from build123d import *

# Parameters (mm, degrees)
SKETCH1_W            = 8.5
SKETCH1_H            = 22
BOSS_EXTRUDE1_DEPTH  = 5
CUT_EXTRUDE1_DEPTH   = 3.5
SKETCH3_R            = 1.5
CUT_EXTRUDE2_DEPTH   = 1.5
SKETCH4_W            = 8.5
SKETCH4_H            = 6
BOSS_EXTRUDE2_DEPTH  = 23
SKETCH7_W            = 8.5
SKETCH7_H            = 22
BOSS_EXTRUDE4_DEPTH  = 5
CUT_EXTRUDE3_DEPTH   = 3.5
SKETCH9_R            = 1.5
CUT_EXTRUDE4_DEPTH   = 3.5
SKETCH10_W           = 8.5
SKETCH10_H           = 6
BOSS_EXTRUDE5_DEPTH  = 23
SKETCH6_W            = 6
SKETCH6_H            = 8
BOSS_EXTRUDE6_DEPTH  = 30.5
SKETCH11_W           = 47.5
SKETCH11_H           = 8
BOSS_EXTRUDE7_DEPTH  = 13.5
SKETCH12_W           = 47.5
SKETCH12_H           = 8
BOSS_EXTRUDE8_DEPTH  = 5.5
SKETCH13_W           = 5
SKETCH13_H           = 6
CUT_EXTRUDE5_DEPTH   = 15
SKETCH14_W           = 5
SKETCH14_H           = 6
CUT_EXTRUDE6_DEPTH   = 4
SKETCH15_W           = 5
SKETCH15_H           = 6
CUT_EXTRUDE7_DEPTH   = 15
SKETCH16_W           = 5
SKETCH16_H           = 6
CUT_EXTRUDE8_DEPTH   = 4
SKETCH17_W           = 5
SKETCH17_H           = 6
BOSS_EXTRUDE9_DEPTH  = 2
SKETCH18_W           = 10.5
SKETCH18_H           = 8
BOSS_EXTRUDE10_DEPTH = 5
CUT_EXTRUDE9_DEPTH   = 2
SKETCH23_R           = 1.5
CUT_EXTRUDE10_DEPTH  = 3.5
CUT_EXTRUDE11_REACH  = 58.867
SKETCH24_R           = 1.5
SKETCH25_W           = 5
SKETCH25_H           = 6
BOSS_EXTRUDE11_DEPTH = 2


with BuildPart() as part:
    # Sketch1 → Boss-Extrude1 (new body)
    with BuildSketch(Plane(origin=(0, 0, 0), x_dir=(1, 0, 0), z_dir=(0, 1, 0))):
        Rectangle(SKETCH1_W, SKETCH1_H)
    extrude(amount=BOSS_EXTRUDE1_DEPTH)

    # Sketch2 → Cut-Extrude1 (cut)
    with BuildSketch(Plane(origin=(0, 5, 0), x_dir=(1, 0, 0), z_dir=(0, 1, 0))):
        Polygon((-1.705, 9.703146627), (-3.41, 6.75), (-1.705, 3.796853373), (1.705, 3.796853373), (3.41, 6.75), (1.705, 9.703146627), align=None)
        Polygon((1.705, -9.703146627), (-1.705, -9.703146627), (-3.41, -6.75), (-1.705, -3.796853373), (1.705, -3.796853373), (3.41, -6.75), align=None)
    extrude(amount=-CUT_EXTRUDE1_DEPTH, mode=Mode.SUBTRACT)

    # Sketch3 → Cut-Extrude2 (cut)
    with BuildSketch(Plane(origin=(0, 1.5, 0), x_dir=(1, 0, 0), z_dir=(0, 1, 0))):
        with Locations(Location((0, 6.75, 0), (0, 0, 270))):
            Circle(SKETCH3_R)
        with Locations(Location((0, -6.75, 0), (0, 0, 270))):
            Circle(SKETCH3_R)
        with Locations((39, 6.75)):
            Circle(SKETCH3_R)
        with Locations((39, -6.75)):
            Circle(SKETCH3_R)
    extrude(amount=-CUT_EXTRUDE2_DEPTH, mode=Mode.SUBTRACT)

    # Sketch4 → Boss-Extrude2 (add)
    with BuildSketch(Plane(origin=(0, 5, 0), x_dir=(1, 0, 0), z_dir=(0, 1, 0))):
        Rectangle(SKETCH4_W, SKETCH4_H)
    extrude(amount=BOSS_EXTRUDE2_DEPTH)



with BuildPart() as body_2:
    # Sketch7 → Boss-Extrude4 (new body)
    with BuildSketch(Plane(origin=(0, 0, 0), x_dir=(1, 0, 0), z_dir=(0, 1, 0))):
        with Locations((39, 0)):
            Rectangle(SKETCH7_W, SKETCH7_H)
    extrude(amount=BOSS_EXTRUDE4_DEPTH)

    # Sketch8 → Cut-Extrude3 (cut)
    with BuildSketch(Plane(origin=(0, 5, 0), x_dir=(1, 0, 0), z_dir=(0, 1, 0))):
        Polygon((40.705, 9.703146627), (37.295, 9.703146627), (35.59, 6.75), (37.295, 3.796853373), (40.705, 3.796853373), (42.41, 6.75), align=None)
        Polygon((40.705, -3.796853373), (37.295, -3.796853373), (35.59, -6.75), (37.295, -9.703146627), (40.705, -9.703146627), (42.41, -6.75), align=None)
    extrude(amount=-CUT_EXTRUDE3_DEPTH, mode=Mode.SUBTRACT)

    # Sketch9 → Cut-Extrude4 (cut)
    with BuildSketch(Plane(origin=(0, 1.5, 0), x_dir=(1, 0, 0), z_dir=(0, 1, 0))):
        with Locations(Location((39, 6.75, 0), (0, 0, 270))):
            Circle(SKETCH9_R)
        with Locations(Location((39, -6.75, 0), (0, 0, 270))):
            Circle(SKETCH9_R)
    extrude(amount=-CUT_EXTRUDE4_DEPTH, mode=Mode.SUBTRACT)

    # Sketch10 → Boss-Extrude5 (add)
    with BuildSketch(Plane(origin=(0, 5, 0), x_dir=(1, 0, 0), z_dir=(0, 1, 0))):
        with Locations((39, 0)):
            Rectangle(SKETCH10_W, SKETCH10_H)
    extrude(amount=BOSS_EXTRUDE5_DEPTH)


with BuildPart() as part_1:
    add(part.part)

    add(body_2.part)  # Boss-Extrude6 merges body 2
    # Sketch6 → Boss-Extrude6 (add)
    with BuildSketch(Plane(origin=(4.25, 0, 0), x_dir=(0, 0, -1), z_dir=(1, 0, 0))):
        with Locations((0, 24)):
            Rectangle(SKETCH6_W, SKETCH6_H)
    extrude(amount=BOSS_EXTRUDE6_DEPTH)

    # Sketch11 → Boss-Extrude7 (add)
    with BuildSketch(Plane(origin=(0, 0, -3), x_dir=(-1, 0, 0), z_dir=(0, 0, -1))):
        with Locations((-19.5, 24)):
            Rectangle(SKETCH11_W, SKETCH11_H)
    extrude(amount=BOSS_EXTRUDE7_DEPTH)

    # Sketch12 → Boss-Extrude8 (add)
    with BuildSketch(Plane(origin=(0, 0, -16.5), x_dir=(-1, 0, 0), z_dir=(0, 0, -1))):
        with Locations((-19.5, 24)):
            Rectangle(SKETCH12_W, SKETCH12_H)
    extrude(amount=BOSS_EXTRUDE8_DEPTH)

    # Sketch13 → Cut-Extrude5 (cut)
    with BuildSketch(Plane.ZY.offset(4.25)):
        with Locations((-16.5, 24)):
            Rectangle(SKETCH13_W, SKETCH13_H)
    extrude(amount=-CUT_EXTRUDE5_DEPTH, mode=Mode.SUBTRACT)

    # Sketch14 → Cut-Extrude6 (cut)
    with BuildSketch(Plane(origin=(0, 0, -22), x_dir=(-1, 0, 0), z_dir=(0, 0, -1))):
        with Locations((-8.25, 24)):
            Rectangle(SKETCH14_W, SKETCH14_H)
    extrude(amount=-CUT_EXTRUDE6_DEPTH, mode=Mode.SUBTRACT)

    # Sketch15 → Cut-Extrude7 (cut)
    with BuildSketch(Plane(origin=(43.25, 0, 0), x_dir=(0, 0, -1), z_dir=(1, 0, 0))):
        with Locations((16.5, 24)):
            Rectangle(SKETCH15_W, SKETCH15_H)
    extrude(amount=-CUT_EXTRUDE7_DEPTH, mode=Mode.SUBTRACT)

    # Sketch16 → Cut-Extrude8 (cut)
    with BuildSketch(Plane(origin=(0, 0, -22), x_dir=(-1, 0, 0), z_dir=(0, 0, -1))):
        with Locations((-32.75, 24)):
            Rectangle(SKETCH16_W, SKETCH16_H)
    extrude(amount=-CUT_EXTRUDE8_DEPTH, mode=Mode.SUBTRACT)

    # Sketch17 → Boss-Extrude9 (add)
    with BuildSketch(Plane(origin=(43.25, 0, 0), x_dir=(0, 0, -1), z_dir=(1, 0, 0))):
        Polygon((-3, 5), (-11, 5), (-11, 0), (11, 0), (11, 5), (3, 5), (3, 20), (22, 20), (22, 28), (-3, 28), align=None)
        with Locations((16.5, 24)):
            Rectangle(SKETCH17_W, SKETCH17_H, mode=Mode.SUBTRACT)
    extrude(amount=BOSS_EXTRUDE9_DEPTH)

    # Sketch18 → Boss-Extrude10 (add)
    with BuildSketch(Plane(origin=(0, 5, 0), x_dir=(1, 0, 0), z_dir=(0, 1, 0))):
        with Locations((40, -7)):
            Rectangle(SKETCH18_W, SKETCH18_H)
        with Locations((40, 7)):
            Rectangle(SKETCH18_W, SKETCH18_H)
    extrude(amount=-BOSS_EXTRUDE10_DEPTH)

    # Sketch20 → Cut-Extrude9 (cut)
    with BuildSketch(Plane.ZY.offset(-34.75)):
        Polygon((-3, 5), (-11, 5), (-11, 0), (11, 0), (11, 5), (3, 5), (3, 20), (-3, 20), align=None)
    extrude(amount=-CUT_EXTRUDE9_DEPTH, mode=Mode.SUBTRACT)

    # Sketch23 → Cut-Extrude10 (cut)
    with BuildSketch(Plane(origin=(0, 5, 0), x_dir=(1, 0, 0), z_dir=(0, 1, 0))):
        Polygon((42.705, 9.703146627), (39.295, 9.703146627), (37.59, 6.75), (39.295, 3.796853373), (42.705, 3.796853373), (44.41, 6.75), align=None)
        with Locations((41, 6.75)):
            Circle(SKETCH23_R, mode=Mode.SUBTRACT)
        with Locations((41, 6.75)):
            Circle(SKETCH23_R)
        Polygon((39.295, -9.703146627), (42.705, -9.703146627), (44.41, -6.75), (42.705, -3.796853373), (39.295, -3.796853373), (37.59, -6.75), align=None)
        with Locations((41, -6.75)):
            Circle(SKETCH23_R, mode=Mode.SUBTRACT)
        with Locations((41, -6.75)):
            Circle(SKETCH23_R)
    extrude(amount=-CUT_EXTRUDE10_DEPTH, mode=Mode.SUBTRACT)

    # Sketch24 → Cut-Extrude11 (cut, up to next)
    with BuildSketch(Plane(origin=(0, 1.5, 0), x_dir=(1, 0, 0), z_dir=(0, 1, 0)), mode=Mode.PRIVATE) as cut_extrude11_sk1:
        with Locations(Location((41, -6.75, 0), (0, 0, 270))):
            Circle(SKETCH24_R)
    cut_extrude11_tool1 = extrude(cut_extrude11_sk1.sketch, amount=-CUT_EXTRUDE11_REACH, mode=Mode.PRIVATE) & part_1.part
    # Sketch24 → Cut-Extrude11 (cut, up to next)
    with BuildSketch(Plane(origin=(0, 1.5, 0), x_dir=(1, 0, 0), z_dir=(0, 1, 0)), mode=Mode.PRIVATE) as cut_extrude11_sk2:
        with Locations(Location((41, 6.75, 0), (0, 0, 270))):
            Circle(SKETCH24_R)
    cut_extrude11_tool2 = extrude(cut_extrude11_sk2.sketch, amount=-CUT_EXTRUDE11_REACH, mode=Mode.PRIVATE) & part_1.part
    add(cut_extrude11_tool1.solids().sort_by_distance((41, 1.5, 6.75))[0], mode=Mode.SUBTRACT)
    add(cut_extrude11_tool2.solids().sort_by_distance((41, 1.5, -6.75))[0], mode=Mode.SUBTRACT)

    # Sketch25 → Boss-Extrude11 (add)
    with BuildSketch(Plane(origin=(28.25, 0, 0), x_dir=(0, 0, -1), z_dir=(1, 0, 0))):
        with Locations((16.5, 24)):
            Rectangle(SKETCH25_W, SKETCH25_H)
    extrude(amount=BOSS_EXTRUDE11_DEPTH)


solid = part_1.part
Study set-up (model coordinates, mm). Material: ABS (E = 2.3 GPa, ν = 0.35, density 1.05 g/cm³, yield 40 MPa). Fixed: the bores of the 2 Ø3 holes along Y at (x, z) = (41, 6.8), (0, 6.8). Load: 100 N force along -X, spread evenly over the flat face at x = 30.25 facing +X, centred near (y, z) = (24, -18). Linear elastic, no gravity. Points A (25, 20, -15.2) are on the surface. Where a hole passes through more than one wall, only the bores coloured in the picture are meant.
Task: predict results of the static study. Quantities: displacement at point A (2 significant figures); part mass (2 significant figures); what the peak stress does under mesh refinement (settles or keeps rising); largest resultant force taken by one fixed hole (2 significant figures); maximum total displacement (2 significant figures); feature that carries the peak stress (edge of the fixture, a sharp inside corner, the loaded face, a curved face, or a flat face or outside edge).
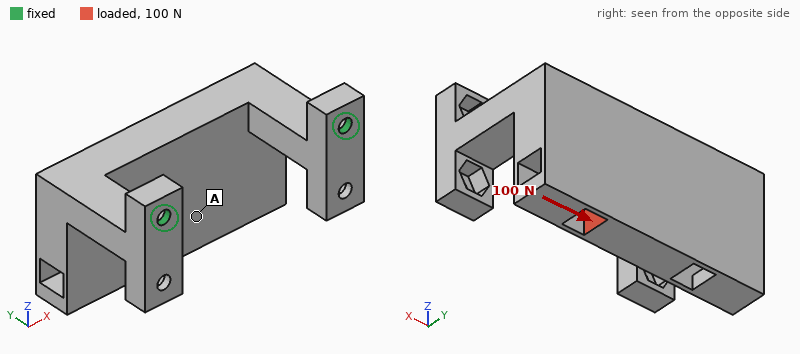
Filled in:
0.53 mm
12 g
keeps rising
81 N
0.70 mm
edge of the fixture
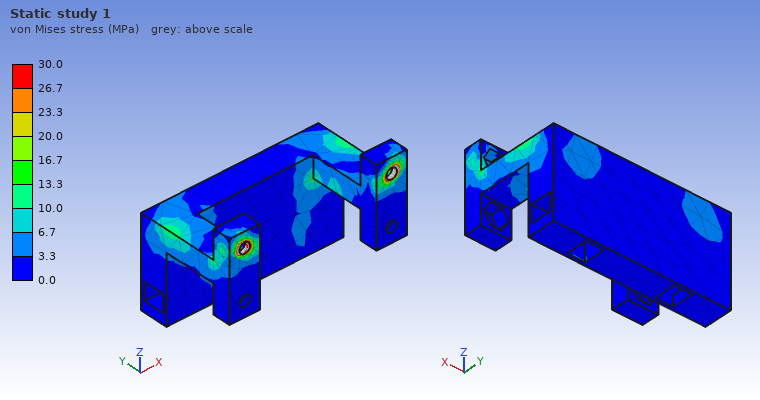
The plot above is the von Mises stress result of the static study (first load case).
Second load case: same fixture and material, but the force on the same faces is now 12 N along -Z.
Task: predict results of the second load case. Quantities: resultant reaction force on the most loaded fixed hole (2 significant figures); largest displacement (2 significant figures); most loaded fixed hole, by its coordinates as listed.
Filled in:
8.3 N
0.71 mm
(41, 6.8)
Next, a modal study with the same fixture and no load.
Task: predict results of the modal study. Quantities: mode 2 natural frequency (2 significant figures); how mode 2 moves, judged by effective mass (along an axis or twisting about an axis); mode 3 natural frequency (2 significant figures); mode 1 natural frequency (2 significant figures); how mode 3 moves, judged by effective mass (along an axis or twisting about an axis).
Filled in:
790 Hz
along X
950 Hz
230 Hz
along X
